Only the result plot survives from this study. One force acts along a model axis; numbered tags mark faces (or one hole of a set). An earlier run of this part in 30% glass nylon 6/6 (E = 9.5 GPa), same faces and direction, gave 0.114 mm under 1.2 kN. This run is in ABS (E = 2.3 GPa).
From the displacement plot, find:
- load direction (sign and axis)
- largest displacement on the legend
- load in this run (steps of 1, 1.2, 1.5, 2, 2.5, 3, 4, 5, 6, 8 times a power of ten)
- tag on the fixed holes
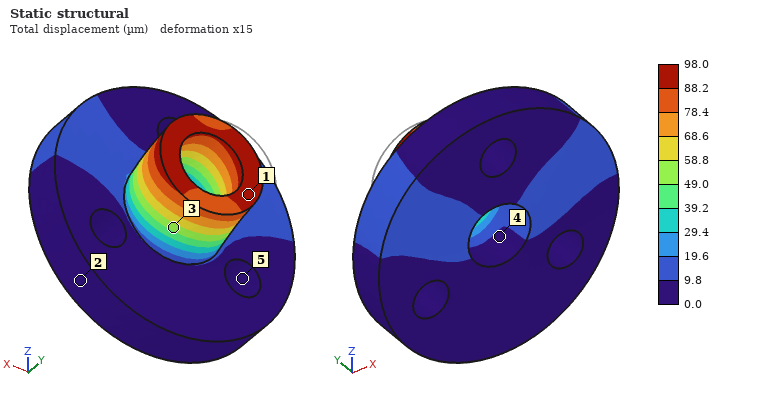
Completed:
+X
98.0 µm
250 N
5
